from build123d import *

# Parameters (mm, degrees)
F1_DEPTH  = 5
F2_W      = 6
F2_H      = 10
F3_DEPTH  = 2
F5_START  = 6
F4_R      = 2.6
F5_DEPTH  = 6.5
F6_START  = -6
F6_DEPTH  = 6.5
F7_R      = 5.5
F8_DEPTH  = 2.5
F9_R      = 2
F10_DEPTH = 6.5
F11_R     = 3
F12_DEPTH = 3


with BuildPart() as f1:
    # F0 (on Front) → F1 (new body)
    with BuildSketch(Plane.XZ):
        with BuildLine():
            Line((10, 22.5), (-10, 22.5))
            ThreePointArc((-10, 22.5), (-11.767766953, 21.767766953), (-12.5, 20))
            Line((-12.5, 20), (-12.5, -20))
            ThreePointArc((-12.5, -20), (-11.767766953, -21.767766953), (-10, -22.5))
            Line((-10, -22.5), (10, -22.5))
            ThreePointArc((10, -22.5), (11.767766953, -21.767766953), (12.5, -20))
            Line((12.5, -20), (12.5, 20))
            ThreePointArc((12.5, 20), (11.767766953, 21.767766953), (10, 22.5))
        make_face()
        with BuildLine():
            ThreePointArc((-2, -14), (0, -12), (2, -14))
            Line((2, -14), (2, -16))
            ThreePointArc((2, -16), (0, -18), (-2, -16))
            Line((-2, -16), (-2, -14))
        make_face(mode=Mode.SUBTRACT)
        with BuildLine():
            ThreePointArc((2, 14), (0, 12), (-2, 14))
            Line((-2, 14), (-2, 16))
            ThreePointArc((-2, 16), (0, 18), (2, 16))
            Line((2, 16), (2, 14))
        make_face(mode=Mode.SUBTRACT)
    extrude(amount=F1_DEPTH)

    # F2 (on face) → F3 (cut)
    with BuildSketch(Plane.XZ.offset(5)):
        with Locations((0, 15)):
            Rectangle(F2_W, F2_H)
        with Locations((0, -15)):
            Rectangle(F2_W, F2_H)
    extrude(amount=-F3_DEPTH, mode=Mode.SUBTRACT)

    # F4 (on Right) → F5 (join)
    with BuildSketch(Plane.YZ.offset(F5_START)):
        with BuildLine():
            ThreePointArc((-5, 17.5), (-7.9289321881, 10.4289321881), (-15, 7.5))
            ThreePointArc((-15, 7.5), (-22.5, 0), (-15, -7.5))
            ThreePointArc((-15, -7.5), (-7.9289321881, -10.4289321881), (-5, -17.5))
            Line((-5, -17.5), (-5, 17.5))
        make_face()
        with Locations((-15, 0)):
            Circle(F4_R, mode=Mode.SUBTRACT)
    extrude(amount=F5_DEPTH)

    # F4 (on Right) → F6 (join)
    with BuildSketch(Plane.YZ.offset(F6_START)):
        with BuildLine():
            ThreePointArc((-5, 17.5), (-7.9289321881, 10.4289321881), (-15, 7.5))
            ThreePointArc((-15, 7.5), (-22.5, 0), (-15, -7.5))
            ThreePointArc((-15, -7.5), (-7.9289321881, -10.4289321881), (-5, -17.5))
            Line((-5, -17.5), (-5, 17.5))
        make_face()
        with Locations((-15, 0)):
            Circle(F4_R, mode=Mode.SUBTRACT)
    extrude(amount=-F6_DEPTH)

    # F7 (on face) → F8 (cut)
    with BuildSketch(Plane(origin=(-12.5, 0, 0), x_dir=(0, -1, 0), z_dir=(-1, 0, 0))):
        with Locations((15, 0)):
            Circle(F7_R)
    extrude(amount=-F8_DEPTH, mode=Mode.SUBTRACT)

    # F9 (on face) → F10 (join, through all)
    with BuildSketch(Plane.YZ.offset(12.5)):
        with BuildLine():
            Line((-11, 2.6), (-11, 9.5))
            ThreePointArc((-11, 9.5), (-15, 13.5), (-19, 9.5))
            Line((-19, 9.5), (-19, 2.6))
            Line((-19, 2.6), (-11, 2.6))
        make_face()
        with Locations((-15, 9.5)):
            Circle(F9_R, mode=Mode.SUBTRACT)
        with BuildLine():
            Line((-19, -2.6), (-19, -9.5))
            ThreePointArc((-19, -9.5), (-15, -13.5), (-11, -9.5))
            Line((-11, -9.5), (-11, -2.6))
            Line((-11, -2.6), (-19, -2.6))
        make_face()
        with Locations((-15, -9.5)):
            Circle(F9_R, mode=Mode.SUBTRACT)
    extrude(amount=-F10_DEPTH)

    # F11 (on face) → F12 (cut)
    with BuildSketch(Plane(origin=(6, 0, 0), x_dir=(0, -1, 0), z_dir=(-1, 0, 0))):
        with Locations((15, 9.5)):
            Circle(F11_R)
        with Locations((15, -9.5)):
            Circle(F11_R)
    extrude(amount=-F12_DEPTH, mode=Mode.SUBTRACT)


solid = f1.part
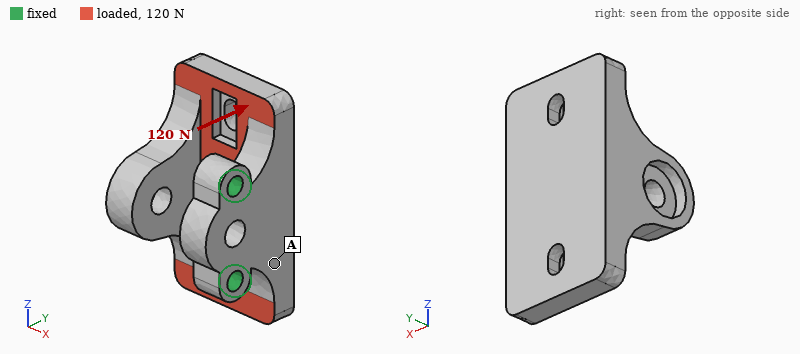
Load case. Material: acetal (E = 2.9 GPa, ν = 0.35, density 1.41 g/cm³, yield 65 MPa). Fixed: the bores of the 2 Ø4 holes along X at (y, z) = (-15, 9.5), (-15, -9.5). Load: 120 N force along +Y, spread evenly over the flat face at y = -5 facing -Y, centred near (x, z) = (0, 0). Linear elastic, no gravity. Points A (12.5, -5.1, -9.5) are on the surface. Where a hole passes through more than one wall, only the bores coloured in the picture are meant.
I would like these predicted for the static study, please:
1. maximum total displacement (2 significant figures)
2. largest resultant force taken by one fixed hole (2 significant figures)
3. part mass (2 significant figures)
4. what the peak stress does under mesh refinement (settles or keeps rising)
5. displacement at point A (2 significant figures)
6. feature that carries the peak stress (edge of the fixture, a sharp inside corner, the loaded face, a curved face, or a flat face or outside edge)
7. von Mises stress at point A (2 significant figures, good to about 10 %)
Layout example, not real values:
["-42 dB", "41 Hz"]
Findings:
["0.63 mm", "60 N", "12 g", "keeps rising", "0.14 mm", "edge of the fixture", "4.5 MPa"]
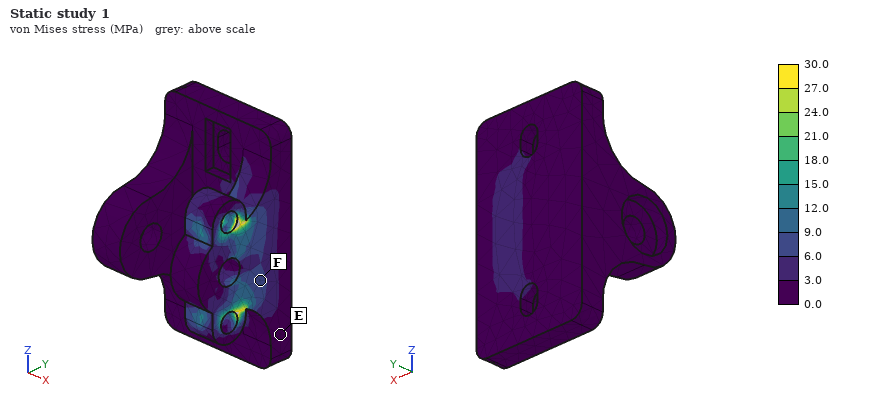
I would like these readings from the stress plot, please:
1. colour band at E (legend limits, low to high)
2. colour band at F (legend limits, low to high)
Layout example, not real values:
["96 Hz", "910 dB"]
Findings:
["0.0 to 3.0 MPa", "6.0 to 9.0 MPa"]
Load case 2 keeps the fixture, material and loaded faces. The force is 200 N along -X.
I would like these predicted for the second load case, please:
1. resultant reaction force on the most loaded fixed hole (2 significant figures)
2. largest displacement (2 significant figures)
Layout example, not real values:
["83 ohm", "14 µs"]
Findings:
["110 N", "0.53 mm"]
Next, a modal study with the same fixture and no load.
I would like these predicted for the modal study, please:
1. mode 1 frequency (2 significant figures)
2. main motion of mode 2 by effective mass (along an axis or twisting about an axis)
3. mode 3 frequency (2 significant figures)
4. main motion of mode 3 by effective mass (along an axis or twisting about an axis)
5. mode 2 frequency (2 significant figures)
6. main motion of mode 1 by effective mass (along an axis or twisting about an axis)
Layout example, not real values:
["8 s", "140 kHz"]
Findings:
["700 Hz", "along Z", "1900 Hz", "along X", "1100 Hz", "along Y"]
